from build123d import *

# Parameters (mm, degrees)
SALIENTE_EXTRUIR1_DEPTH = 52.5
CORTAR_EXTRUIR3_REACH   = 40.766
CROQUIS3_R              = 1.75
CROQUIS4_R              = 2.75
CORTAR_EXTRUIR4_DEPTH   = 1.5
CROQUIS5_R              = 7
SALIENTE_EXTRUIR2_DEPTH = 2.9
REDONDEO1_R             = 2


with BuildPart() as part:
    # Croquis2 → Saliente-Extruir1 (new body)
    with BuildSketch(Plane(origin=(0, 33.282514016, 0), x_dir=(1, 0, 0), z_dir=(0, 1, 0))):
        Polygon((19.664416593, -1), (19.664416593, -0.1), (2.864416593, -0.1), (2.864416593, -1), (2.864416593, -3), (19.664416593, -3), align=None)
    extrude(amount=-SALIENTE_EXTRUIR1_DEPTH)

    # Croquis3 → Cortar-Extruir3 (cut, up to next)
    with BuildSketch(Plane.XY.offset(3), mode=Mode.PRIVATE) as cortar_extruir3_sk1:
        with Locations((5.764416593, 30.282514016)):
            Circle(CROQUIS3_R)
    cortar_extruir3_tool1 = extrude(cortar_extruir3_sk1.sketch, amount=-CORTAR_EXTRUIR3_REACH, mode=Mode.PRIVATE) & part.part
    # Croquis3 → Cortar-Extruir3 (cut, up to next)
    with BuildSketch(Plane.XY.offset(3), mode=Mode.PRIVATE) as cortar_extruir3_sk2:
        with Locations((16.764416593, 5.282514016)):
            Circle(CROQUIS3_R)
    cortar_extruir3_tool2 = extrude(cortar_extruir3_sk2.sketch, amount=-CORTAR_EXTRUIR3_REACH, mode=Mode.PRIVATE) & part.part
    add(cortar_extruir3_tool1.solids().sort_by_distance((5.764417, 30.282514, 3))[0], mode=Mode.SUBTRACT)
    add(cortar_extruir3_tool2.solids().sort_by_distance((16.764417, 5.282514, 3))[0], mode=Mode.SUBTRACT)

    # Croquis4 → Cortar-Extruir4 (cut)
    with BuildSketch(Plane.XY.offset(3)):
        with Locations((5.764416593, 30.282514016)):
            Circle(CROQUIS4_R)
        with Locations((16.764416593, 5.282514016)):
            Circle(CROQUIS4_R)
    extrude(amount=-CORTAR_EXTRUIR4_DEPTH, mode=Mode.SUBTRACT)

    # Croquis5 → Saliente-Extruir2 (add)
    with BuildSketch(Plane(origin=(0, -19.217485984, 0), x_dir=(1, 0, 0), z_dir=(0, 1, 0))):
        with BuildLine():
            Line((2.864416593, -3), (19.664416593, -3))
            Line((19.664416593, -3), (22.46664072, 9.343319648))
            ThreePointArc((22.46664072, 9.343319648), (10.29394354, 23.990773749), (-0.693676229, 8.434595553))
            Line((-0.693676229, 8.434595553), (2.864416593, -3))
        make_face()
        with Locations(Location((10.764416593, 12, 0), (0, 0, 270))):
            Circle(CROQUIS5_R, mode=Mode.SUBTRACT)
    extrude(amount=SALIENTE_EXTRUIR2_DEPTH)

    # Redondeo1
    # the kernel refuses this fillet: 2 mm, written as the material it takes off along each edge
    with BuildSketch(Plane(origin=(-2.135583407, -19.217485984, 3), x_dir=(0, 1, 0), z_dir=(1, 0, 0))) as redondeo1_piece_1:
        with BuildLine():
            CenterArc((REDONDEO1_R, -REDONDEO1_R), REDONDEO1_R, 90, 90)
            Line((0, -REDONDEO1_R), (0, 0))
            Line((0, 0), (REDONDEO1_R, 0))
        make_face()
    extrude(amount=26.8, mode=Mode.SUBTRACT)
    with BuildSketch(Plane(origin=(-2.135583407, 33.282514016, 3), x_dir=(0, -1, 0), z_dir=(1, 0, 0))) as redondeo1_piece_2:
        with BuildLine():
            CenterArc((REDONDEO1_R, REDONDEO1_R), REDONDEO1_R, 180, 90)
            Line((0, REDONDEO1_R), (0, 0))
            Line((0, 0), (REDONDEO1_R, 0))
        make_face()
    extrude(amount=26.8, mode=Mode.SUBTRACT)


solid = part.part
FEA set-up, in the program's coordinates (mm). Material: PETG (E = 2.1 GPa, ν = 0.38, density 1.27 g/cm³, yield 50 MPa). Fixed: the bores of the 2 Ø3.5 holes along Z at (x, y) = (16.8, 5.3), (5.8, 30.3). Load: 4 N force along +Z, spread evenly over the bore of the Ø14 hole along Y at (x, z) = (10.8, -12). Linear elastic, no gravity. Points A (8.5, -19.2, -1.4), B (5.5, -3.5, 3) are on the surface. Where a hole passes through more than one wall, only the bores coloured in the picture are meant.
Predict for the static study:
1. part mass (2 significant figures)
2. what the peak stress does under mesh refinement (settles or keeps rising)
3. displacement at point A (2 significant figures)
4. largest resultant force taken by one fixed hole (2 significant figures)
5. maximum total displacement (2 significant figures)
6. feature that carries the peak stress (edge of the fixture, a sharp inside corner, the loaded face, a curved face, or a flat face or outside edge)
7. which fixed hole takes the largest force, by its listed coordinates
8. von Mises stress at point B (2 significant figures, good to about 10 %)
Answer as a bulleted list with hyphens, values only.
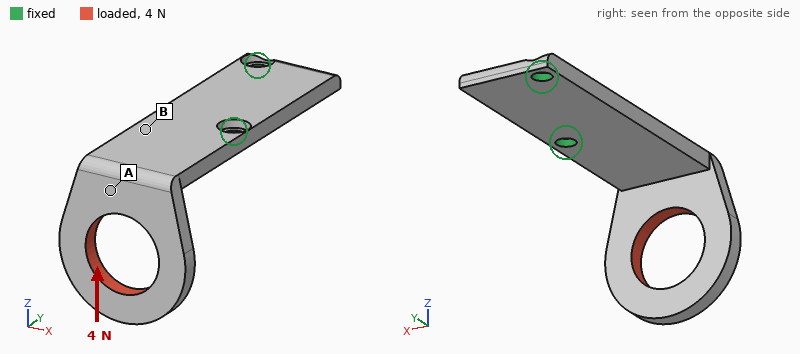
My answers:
- 4.3 g
- keeps rising
- 0.40 mm
- 7.3 N
- 0.65 mm
- edge of the fixture
- (16.8, 5.3)
- 2.3 MPa
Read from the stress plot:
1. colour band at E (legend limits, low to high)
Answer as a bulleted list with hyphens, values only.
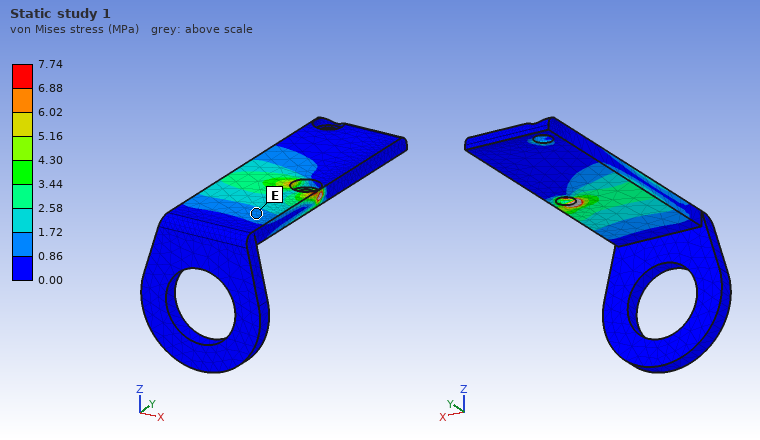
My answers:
- 0.86 to 1.72 MPa
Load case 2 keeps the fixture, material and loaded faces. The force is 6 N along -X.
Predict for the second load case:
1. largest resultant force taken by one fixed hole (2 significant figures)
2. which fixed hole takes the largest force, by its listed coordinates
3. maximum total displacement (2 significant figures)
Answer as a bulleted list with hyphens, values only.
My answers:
- 10 N
- (16.8, 5.3)
- 0.66 mm
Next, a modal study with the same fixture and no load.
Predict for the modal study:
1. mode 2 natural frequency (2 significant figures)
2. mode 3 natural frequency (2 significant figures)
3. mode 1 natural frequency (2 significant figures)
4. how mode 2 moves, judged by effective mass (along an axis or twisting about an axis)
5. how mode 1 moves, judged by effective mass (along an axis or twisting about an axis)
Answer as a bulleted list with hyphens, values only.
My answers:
- 490 Hz
- 890 Hz
- 320 Hz
- along X
- along Z
